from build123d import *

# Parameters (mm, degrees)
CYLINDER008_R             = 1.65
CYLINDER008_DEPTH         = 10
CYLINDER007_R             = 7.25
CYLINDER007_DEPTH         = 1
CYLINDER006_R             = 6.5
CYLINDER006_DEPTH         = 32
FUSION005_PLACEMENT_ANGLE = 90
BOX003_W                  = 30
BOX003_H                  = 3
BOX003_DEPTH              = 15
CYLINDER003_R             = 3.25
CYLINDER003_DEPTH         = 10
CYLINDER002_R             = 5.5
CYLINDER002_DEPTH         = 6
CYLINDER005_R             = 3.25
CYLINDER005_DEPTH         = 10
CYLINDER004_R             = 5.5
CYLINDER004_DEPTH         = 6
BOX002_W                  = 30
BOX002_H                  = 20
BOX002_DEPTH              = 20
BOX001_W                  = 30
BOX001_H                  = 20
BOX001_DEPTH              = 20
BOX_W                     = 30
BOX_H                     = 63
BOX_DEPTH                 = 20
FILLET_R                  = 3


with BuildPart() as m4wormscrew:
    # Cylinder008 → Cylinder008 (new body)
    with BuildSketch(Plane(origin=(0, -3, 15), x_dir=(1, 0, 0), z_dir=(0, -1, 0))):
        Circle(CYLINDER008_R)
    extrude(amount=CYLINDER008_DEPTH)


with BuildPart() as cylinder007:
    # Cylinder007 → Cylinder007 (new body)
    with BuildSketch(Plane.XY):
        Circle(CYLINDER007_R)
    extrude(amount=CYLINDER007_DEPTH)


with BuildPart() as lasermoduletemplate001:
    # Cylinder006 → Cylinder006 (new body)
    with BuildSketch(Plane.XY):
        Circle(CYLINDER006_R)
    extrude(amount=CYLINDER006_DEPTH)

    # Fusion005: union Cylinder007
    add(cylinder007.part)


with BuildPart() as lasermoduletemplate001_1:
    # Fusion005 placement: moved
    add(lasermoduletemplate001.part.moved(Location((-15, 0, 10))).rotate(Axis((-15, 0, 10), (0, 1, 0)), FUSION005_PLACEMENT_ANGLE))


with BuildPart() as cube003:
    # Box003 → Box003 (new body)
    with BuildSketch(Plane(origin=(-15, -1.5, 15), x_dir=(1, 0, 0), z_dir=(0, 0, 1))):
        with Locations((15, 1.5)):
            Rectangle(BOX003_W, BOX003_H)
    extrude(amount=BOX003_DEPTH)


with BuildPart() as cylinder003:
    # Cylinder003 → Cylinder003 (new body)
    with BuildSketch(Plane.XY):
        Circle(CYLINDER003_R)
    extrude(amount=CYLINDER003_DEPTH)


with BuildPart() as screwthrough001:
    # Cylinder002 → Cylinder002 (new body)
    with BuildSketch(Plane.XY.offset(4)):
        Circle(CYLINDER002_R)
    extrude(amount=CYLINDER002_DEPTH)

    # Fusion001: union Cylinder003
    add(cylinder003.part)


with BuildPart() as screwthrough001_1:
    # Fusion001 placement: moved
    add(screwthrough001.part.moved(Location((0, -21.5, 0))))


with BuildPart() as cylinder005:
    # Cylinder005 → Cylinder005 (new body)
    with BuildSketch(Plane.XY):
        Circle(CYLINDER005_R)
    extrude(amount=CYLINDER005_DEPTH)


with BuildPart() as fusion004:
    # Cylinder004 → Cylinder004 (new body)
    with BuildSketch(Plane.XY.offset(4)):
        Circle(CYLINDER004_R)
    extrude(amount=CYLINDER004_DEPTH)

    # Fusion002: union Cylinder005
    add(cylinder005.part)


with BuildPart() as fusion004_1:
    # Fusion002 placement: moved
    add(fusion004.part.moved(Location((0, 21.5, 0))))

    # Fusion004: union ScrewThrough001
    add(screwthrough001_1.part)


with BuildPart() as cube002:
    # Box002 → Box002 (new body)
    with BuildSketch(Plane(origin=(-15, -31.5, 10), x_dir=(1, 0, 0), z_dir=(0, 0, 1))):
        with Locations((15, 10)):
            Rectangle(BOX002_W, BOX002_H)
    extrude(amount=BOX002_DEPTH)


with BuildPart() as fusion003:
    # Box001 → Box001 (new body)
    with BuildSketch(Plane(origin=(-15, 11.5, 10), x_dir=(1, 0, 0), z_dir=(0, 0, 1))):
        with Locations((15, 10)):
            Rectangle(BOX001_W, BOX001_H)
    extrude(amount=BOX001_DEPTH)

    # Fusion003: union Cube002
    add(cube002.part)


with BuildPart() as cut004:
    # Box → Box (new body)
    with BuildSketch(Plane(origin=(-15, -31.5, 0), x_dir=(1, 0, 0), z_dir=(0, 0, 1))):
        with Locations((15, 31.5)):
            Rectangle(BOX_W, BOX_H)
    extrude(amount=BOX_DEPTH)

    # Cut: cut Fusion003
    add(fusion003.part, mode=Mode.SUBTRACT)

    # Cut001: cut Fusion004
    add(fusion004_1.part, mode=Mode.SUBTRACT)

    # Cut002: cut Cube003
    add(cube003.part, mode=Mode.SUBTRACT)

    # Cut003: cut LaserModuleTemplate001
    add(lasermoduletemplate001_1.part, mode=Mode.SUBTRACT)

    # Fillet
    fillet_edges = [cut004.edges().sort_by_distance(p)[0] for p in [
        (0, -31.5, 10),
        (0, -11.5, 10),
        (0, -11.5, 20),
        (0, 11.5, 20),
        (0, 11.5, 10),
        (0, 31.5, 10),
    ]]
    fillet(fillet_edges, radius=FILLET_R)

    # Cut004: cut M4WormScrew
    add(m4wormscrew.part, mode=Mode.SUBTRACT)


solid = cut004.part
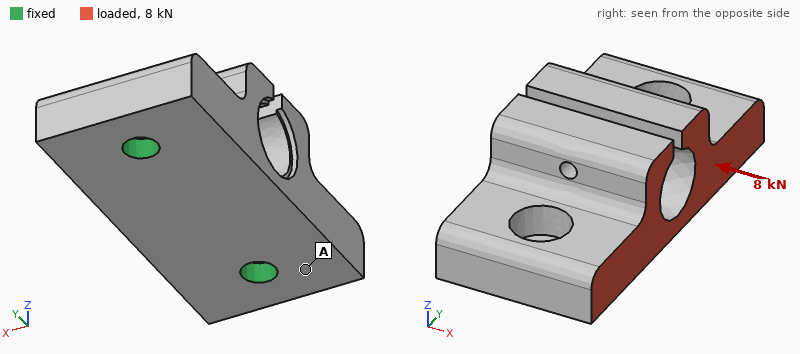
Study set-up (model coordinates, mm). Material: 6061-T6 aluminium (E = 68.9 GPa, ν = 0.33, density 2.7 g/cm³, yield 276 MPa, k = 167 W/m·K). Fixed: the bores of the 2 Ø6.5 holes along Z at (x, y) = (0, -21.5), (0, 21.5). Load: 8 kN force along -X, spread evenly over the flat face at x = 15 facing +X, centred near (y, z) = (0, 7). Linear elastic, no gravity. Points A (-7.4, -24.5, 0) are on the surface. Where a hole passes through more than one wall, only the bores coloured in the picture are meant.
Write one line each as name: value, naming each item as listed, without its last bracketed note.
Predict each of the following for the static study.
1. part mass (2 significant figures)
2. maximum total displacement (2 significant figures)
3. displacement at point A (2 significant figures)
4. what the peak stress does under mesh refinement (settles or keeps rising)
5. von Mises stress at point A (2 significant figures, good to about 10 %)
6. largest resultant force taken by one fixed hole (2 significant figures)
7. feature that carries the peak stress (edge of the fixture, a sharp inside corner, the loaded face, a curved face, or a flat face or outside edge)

part mass: 54 g
maximum total displacement: 83 µm
displacement at point A: 16 µm
what the peak stress does under mesh refinement: keeps rising
von Mises stress at point A: 34 MPa
largest resultant force taken by one fixed hole: 4.0 kN
feature that carries the peak stress: edge of the fixture
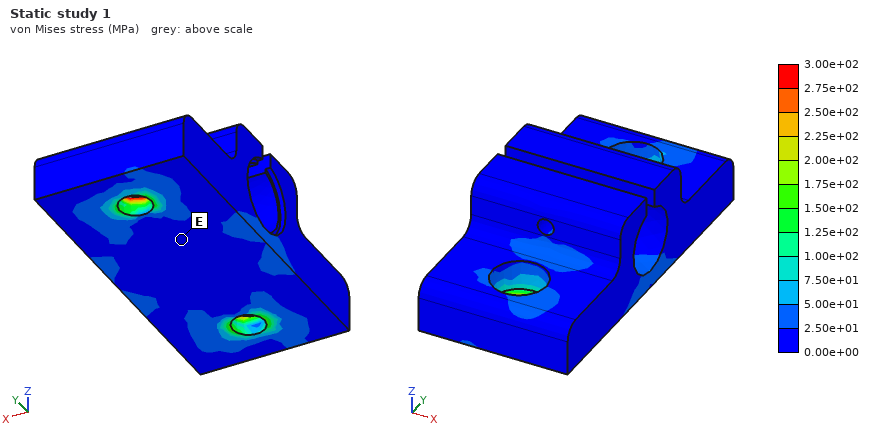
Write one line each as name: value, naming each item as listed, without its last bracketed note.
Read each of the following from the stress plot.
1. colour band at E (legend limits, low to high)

colour band at E: 0.00e+00 to 2.50e+01 MPa
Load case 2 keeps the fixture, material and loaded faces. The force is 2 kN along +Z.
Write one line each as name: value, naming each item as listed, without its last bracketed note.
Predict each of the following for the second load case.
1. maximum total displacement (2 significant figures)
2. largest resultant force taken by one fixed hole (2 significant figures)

maximum total displacement: 69 µm
largest resultant force taken by one fixed hole: 1.0 kN
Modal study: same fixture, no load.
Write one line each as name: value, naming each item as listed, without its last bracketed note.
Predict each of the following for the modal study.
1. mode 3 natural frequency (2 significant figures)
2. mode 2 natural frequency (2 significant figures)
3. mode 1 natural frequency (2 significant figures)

mode 3 natural frequency: 11 kHz
mode 2 natural frequency: 7000 Hz
mode 1 natural frequency: 6700 Hz
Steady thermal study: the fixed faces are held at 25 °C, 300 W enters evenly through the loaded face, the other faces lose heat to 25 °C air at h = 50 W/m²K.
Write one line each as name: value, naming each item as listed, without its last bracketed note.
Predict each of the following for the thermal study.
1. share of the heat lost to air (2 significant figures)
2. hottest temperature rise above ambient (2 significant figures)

share of the heat lost to air: 4.7 %
hottest temperature rise above ambient: 80 K
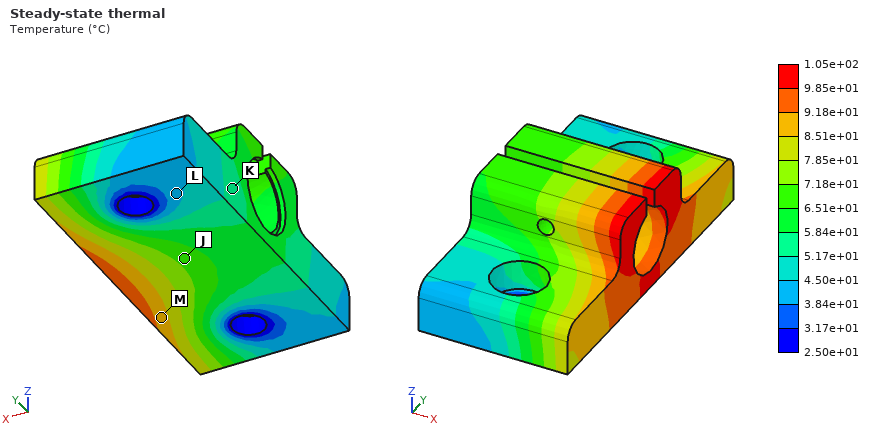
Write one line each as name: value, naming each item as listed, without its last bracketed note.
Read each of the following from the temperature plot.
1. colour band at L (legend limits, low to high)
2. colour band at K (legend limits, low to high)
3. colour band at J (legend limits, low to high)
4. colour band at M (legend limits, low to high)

colour band at L: 3.84e+01 to 4.50e+01 °C
colour band at K: 5.17e+01 to 5.84e+01 °C
colour band at J: 6.51e+01 to 7.18e+01 °C
colour band at M: 8.51e+01 to 9.18e+01 °C
